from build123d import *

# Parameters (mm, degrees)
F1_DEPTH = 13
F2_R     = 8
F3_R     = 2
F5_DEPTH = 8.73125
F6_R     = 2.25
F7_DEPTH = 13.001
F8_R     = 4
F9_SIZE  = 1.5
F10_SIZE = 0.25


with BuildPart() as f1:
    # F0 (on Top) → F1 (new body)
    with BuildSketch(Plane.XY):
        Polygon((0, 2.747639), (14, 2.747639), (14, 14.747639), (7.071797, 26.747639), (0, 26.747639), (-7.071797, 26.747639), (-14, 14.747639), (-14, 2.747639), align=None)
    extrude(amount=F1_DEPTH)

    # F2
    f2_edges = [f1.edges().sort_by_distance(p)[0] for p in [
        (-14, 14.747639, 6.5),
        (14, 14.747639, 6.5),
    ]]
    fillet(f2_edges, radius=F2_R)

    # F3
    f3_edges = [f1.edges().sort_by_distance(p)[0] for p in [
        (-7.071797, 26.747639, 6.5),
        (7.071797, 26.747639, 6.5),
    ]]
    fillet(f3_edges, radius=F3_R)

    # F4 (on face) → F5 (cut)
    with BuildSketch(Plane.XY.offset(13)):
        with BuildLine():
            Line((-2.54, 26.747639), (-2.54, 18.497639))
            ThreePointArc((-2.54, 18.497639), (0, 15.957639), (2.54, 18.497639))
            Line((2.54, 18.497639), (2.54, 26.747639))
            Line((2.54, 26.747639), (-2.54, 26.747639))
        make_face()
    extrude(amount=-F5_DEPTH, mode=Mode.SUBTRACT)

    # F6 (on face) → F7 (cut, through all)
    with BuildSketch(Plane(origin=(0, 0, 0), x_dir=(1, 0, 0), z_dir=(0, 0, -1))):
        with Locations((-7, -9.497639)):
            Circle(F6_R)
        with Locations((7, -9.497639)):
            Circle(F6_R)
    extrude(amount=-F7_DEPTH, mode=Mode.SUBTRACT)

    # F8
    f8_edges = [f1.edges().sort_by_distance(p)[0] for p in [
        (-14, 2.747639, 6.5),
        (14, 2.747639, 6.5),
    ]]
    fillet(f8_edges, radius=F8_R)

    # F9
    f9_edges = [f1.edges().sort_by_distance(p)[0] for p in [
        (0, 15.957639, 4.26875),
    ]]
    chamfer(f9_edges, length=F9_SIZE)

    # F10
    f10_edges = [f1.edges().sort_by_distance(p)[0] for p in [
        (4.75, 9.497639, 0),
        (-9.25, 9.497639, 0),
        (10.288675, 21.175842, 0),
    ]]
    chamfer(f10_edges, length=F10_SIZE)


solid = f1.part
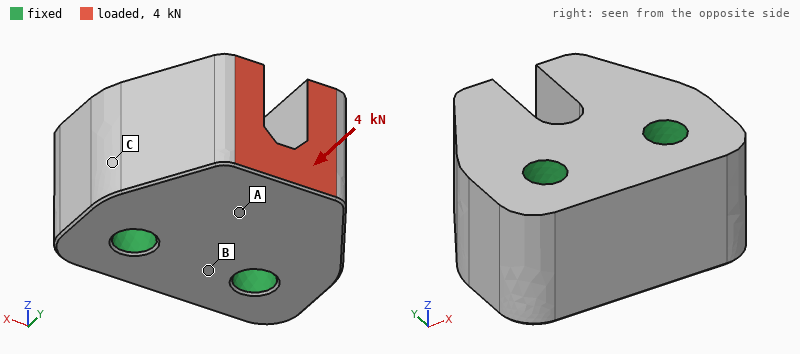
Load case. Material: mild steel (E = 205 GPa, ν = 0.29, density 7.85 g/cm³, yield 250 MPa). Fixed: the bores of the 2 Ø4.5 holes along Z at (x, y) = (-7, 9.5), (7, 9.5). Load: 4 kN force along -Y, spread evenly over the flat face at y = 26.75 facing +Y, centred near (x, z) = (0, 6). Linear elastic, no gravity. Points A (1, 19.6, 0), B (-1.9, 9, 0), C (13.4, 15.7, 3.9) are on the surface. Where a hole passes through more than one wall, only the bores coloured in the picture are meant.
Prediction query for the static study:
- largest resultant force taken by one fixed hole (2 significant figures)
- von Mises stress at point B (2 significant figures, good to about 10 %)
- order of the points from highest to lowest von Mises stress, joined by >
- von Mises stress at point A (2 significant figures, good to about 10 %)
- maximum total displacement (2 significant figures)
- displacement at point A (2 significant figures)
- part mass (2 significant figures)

2.1 kN
9.4 MPa
A > B > C
31 MPa
2.9 µm
1.4 µm
53 g
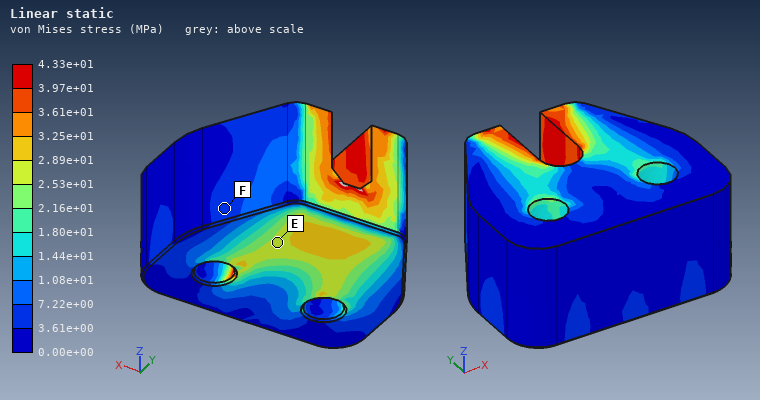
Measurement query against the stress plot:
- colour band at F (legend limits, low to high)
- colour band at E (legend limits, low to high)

3.61e+00 to 7.22e+00 MPa
2.53e+01 to 2.89e+01 MPa
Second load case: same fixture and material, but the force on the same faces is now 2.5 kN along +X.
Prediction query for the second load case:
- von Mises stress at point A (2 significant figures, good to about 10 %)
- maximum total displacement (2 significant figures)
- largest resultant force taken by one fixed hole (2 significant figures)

23 MPa
6.9 µm
2.6 kN
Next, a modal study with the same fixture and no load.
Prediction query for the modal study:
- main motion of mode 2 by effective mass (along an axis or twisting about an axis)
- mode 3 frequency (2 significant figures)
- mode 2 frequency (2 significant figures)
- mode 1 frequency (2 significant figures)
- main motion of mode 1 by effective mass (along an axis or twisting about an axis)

along X
49 kHz
40 kHz
34 kHz
along Z
